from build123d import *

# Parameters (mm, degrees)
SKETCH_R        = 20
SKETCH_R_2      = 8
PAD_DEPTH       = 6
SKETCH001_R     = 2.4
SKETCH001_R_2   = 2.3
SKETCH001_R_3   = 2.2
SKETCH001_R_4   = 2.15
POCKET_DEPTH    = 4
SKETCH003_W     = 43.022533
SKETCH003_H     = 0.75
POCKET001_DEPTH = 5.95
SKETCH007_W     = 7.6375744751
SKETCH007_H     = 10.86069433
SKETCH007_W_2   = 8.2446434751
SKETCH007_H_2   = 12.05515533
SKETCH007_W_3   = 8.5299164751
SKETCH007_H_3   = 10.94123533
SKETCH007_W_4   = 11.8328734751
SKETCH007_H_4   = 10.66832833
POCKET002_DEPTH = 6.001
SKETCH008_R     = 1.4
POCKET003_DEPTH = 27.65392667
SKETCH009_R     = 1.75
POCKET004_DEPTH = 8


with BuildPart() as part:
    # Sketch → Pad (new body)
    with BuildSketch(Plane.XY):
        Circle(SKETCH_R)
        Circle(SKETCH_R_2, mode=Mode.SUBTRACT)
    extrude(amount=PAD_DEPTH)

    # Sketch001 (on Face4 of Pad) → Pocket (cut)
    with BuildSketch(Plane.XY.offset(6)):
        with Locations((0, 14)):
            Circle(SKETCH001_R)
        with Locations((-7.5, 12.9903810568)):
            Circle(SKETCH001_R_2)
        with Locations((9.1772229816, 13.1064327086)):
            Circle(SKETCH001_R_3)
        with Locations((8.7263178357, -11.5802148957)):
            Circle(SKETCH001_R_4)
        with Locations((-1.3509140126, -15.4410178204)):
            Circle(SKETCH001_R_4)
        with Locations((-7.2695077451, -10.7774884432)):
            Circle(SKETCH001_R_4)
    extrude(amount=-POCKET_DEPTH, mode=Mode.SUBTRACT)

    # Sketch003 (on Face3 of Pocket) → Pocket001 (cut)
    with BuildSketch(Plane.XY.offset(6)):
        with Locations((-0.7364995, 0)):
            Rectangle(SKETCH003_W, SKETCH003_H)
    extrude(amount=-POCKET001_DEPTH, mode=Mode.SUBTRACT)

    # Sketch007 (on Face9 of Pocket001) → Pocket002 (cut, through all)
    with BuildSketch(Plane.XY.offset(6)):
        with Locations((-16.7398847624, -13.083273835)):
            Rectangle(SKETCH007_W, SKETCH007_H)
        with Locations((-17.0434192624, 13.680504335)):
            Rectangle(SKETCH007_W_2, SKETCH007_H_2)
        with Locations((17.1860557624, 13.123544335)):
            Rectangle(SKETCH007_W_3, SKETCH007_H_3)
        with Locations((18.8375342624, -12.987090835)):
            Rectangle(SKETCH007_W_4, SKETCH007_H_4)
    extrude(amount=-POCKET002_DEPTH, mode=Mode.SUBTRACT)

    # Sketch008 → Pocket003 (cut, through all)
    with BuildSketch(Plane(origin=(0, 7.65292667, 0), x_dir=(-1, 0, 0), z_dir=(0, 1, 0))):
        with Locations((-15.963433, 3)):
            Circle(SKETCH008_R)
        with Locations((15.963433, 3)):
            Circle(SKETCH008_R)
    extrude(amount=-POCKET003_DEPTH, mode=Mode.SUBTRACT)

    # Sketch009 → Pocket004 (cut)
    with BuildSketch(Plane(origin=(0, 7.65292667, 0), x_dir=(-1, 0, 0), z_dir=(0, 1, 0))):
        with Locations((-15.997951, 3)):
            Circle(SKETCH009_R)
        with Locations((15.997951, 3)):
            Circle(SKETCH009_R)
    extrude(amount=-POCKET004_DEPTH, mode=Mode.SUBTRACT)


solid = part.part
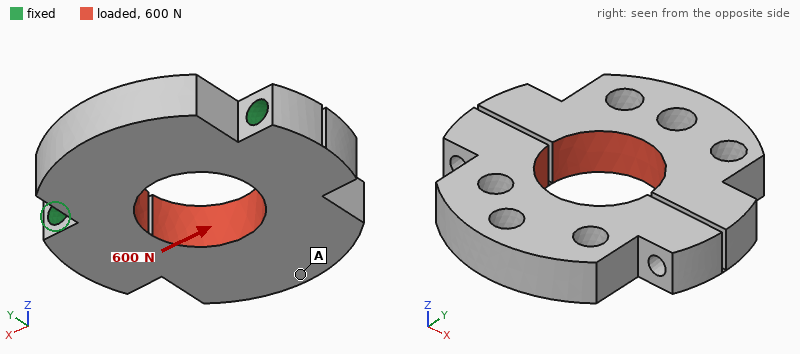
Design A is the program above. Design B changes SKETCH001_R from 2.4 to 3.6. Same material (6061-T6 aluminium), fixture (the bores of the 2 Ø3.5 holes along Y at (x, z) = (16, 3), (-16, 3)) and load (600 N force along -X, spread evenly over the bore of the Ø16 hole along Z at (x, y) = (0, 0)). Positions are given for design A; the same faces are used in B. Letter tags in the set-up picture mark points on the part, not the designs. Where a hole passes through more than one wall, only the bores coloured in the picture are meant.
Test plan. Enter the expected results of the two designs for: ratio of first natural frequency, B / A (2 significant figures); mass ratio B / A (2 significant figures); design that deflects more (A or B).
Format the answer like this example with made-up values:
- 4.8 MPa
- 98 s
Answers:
- 1.0
- 0.98
- B
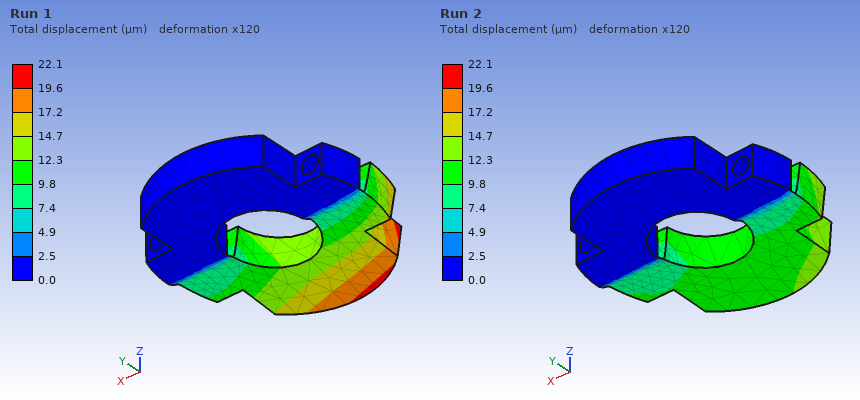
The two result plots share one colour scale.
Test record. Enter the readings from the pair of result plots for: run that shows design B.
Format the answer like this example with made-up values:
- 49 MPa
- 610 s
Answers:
- Run 1
